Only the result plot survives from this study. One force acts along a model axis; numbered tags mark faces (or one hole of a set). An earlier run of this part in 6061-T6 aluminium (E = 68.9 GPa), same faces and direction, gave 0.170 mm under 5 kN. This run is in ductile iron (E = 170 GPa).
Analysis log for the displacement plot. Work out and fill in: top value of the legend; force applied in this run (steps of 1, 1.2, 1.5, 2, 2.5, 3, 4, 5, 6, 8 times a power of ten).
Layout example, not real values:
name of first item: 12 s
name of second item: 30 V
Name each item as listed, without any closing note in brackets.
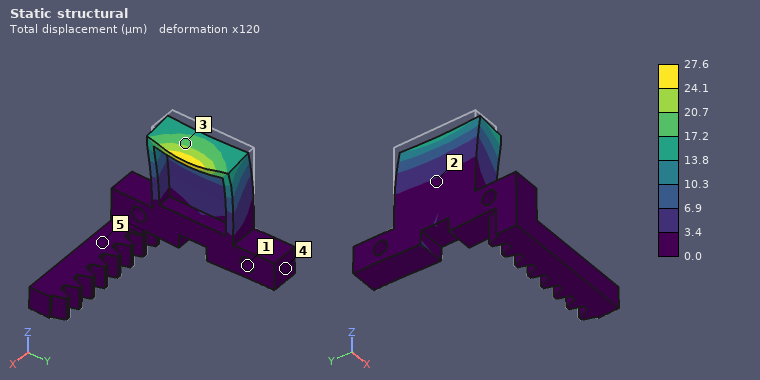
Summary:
top value of the legend: 27.6 µm
force applied in this run: 2 kN
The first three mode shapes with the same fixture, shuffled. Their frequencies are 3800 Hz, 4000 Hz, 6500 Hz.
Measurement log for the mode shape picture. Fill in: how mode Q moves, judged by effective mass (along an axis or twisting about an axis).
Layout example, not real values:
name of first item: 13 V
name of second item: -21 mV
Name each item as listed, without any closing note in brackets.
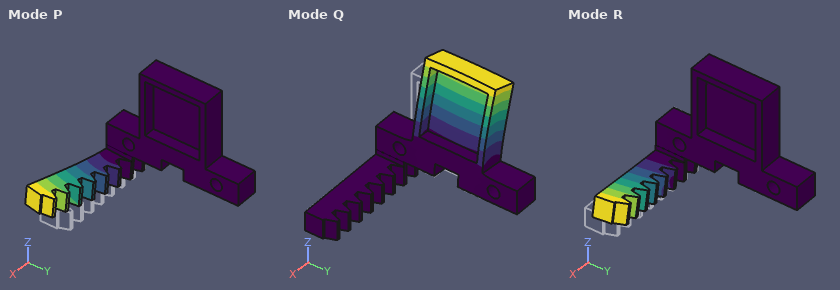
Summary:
how mode Q moves, judged by effective mass: along X
